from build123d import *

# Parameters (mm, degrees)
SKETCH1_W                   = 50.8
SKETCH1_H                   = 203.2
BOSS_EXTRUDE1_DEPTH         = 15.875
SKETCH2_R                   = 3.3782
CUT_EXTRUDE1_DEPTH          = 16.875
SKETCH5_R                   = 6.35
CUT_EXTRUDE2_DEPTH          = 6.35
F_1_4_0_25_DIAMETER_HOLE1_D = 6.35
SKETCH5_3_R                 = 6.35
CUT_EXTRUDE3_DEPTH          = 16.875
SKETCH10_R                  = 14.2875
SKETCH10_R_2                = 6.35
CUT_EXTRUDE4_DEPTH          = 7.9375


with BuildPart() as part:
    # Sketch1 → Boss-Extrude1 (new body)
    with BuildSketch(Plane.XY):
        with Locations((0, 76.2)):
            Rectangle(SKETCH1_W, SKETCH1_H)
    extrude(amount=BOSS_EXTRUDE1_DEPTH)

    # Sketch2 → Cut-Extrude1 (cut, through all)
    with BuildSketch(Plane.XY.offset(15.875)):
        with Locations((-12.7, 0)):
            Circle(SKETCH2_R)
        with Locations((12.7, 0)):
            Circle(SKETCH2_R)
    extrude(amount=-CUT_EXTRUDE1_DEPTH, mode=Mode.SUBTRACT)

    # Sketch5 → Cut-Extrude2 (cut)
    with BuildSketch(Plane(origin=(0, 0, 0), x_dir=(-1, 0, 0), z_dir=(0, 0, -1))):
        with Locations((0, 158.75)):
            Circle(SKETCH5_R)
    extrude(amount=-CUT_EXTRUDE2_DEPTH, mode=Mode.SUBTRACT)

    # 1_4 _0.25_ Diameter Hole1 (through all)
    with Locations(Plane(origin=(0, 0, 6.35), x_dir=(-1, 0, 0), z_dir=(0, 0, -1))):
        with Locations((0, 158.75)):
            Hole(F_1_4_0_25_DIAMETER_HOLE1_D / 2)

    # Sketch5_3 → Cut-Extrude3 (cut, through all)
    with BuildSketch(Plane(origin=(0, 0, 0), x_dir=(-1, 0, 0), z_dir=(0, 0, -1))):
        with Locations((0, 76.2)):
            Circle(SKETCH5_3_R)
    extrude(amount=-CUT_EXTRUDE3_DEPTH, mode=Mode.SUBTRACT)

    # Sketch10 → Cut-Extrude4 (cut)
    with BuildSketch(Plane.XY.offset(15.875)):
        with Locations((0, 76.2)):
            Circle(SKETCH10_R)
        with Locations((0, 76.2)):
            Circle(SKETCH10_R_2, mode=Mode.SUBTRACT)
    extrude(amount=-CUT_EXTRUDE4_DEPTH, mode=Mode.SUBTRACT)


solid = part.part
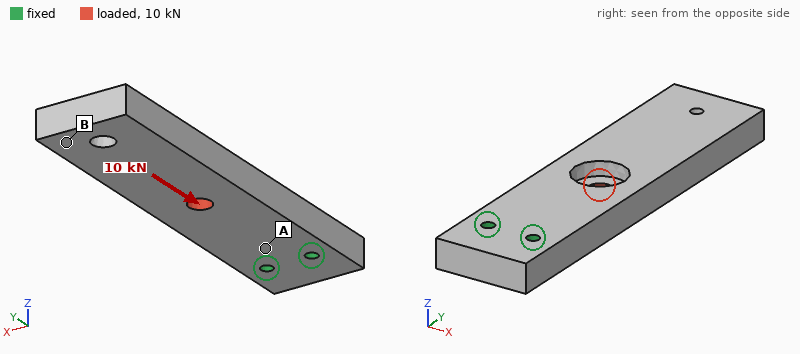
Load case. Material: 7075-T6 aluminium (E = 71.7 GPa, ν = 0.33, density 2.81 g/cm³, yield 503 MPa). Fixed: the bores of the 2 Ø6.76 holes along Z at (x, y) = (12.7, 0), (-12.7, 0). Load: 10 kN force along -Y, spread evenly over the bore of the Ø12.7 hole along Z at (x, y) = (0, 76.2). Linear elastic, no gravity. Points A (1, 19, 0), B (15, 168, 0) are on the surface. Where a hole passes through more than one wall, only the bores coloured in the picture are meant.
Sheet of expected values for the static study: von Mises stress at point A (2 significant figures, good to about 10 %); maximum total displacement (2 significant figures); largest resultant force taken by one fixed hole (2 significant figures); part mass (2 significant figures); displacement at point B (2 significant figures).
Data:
29 MPa
0.35 mm
5.0 kN
440 g
0.33 mm
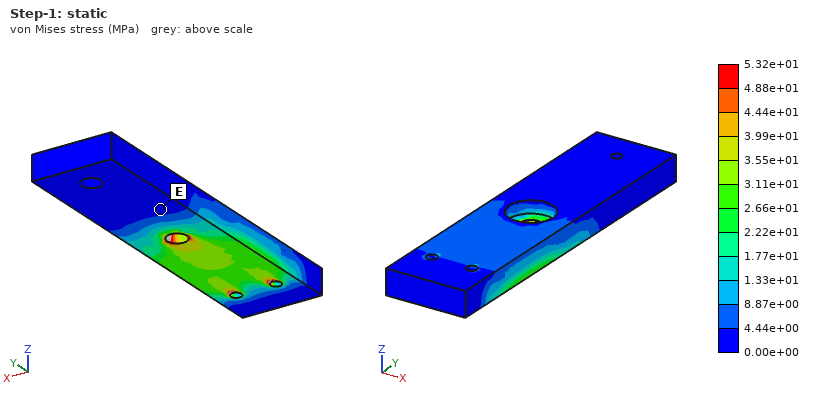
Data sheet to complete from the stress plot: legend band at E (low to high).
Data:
0.00e+00 to 4.44e+00 MPa
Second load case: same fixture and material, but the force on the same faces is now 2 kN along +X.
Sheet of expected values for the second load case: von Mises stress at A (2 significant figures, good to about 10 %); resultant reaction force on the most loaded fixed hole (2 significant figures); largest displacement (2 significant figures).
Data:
12 MPa
5.3 kN
98 µm
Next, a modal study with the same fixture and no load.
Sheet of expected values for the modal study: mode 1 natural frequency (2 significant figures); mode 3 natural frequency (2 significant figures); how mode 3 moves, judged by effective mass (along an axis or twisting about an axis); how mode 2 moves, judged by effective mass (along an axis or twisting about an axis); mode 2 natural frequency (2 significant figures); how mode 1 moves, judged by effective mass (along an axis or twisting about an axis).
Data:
400 Hz
2300 Hz
twisting about Y
along X
1200 Hz
along Z
